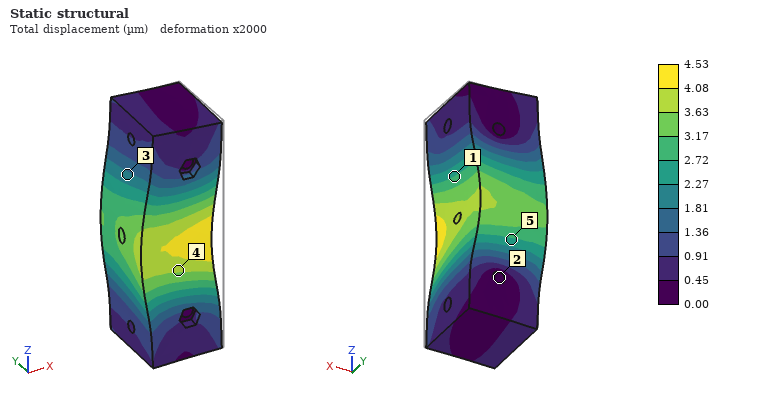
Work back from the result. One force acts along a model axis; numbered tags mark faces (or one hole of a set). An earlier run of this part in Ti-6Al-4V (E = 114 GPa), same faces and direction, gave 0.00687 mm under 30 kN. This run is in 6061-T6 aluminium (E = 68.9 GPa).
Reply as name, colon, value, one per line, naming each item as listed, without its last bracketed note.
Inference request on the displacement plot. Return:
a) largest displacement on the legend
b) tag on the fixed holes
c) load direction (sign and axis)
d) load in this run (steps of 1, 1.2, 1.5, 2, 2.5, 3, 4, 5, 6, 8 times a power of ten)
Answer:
largest displacement on the legend: 4.53 µm
tag on the fixed holes: 2
load direction: -X
load in this run: 12 kN
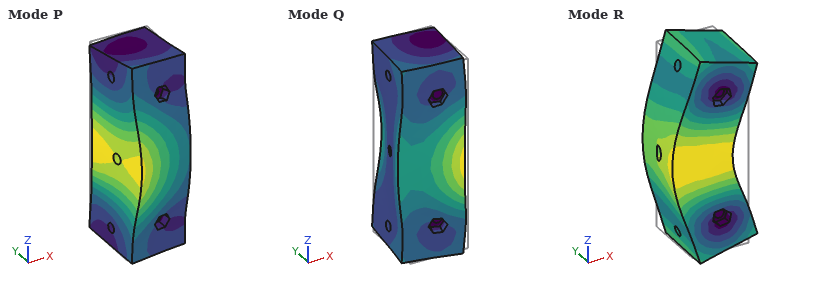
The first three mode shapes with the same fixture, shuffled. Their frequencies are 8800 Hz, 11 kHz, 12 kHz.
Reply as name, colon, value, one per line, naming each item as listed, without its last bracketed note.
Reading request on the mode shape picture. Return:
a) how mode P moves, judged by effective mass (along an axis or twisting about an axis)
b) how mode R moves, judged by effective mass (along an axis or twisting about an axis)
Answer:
how mode P moves, judged by effective mass: along Y
how mode R moves, judged by effective mass: along X
